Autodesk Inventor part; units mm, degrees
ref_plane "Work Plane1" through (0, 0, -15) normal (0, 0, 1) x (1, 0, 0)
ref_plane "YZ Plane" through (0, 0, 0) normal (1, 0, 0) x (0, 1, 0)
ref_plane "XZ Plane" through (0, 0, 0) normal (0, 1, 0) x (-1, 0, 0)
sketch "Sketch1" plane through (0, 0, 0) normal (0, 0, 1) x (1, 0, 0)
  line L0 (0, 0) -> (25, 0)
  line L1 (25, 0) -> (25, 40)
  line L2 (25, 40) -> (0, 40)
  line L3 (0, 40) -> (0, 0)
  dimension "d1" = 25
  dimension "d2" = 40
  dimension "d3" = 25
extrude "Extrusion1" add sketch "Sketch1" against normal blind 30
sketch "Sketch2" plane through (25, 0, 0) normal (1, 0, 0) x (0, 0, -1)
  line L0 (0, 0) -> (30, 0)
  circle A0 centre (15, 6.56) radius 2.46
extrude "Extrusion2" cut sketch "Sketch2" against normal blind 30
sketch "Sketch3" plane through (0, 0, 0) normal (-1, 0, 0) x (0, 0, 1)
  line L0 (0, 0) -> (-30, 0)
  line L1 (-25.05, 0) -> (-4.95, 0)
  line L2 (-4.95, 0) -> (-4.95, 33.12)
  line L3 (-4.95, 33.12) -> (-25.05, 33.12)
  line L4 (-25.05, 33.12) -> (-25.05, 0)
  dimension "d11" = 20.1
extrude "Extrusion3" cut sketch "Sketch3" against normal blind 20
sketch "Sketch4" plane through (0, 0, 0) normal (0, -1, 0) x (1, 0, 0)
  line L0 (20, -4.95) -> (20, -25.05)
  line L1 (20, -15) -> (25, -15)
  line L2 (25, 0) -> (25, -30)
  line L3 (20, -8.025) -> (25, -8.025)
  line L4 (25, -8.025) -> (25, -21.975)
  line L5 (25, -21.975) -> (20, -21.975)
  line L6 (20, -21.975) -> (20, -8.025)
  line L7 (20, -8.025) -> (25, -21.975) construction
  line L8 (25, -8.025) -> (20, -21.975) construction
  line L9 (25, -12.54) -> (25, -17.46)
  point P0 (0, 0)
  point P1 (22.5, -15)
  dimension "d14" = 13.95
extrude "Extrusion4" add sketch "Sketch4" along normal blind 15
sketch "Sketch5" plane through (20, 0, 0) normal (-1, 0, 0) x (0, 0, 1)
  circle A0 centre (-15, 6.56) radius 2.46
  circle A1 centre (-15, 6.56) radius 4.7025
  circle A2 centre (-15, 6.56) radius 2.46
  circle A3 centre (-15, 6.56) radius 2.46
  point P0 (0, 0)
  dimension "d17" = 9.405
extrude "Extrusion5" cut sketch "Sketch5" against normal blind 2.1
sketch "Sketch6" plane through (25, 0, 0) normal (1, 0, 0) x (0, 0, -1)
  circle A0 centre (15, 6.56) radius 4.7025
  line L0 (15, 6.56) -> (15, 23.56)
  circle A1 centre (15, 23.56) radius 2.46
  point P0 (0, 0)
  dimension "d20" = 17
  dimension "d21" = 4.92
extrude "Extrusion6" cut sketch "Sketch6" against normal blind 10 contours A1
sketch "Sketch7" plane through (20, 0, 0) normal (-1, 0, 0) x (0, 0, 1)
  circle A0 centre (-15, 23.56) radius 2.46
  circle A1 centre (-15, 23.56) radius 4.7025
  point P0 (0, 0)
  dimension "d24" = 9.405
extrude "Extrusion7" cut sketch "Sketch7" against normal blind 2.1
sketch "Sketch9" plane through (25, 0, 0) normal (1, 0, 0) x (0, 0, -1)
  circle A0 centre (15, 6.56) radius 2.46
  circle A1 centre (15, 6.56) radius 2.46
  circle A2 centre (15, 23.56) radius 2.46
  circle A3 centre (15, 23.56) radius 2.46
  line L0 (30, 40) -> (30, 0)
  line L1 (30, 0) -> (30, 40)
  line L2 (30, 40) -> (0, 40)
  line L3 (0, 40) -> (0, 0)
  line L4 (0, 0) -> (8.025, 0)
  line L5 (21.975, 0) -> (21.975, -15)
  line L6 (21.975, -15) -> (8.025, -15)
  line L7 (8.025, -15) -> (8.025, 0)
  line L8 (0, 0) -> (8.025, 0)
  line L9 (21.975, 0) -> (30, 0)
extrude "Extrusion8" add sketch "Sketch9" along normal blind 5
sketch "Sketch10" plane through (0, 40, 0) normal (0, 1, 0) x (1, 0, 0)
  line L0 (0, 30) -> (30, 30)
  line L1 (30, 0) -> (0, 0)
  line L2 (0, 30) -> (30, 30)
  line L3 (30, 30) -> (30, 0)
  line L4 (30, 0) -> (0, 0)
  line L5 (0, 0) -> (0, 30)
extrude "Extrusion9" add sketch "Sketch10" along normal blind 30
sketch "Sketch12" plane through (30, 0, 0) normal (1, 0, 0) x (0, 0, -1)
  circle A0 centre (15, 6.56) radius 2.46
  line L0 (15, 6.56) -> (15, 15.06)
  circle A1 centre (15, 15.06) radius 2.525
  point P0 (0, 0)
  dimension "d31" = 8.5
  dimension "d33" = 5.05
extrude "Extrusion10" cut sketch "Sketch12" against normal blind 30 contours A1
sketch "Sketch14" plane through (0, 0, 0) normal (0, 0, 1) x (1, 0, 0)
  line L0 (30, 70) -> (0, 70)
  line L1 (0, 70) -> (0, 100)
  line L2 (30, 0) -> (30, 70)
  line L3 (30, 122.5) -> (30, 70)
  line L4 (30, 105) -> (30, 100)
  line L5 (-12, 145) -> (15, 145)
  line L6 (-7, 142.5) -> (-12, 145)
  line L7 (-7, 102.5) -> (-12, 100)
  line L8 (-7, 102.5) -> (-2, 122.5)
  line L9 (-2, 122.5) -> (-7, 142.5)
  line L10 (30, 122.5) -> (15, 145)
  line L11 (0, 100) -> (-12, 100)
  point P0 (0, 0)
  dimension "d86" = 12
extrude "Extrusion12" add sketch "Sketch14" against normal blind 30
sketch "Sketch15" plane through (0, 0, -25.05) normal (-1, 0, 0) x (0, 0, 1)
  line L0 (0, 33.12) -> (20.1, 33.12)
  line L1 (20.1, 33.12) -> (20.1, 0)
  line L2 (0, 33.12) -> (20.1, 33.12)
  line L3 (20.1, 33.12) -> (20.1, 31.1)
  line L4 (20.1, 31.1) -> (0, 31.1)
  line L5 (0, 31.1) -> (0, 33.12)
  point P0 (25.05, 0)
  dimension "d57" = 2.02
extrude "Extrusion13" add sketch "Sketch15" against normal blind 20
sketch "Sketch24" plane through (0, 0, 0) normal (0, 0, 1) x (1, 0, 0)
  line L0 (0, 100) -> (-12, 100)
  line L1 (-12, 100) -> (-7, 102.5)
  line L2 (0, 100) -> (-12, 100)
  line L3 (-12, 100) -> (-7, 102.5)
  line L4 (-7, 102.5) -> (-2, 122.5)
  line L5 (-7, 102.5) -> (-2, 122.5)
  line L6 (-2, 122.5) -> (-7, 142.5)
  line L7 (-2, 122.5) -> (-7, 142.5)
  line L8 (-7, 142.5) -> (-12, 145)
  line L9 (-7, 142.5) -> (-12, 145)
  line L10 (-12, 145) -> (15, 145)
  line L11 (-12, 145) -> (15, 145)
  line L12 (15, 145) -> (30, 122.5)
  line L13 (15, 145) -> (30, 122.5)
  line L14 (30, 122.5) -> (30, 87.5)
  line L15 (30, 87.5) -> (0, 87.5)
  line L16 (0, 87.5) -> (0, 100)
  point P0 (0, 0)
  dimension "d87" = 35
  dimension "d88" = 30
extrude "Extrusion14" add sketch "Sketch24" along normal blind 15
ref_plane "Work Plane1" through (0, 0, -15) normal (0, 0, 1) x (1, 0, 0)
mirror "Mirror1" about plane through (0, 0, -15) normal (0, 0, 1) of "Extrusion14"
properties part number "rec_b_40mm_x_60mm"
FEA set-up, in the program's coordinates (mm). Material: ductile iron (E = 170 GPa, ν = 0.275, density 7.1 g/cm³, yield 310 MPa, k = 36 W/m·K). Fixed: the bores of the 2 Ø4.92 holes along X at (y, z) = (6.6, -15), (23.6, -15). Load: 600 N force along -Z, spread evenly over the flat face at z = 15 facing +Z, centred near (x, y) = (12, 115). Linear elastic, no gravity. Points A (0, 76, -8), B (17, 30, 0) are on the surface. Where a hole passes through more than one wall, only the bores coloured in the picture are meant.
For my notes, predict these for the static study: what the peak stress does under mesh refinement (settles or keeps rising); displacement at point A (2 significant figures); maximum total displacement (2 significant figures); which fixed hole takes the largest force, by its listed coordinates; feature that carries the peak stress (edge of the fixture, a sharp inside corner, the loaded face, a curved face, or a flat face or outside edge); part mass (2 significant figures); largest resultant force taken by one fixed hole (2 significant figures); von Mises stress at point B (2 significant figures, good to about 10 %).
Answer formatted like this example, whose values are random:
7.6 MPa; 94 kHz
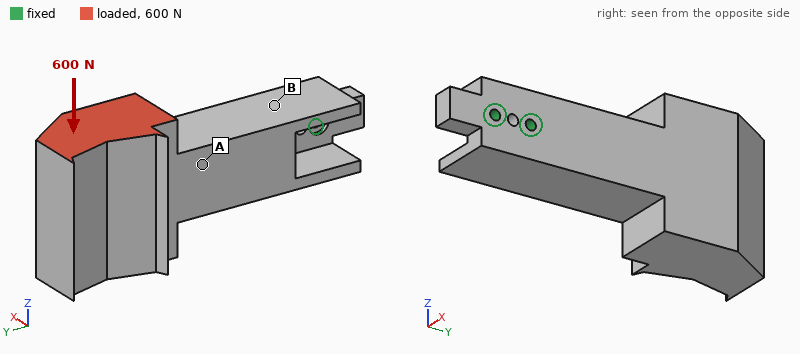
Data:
keeps rising; 23 µm; 60 µm; (23.6, -15); edge of the fixture; 1.2 kg; 2.9 kN; 19 MPa
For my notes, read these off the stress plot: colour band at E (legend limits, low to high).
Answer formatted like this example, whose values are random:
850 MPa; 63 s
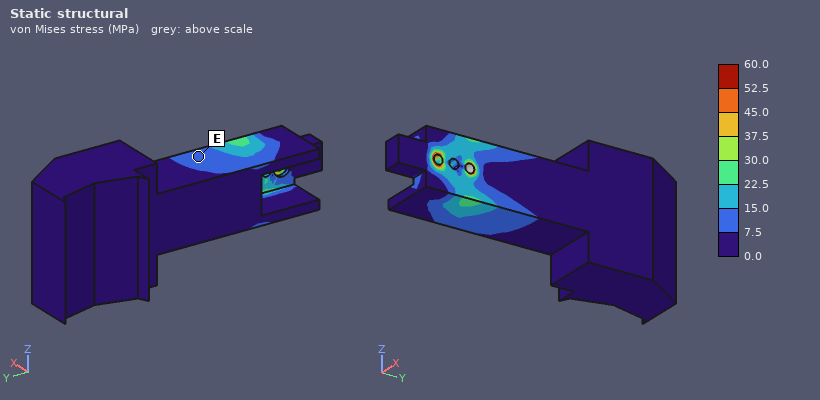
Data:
7.5 to 15.0 MPa
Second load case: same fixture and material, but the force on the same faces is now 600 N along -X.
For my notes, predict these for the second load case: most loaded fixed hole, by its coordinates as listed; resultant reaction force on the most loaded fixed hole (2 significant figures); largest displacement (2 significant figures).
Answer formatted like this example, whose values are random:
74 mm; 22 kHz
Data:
(23.6, -15); 2.8 kN; 95 µm
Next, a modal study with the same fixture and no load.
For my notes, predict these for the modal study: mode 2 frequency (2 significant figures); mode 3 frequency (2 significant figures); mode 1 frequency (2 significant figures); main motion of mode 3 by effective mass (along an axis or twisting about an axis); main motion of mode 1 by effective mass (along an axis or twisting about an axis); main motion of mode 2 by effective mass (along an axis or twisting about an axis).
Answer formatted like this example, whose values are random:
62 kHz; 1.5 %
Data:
640 Hz; 1600 Hz; 560 Hz; twisting about Y; along X; along Z
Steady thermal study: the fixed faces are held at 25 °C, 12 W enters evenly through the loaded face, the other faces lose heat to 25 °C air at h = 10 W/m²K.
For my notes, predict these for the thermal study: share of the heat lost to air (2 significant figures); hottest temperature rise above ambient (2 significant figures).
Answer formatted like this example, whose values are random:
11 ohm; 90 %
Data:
38 %; 31 K
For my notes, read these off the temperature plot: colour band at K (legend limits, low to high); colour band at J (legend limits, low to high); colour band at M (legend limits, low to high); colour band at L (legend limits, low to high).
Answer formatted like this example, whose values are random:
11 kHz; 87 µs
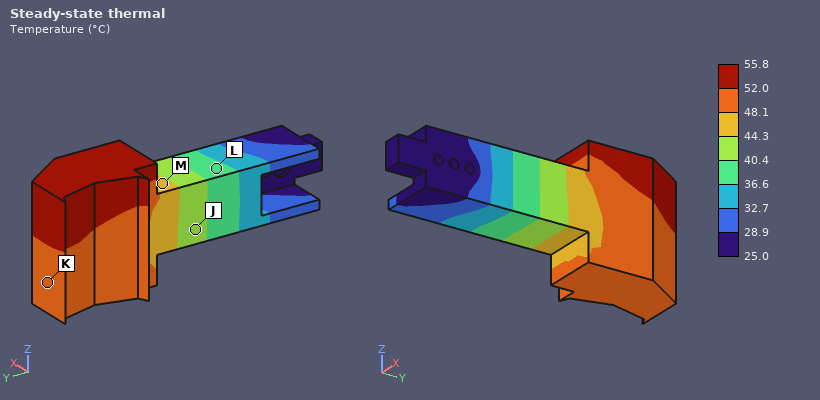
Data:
48.1 to 52.0 °C; 40.4 to 44.3 °C; 44.3 to 48.1 °C; 36.6 to 40.4 °C
